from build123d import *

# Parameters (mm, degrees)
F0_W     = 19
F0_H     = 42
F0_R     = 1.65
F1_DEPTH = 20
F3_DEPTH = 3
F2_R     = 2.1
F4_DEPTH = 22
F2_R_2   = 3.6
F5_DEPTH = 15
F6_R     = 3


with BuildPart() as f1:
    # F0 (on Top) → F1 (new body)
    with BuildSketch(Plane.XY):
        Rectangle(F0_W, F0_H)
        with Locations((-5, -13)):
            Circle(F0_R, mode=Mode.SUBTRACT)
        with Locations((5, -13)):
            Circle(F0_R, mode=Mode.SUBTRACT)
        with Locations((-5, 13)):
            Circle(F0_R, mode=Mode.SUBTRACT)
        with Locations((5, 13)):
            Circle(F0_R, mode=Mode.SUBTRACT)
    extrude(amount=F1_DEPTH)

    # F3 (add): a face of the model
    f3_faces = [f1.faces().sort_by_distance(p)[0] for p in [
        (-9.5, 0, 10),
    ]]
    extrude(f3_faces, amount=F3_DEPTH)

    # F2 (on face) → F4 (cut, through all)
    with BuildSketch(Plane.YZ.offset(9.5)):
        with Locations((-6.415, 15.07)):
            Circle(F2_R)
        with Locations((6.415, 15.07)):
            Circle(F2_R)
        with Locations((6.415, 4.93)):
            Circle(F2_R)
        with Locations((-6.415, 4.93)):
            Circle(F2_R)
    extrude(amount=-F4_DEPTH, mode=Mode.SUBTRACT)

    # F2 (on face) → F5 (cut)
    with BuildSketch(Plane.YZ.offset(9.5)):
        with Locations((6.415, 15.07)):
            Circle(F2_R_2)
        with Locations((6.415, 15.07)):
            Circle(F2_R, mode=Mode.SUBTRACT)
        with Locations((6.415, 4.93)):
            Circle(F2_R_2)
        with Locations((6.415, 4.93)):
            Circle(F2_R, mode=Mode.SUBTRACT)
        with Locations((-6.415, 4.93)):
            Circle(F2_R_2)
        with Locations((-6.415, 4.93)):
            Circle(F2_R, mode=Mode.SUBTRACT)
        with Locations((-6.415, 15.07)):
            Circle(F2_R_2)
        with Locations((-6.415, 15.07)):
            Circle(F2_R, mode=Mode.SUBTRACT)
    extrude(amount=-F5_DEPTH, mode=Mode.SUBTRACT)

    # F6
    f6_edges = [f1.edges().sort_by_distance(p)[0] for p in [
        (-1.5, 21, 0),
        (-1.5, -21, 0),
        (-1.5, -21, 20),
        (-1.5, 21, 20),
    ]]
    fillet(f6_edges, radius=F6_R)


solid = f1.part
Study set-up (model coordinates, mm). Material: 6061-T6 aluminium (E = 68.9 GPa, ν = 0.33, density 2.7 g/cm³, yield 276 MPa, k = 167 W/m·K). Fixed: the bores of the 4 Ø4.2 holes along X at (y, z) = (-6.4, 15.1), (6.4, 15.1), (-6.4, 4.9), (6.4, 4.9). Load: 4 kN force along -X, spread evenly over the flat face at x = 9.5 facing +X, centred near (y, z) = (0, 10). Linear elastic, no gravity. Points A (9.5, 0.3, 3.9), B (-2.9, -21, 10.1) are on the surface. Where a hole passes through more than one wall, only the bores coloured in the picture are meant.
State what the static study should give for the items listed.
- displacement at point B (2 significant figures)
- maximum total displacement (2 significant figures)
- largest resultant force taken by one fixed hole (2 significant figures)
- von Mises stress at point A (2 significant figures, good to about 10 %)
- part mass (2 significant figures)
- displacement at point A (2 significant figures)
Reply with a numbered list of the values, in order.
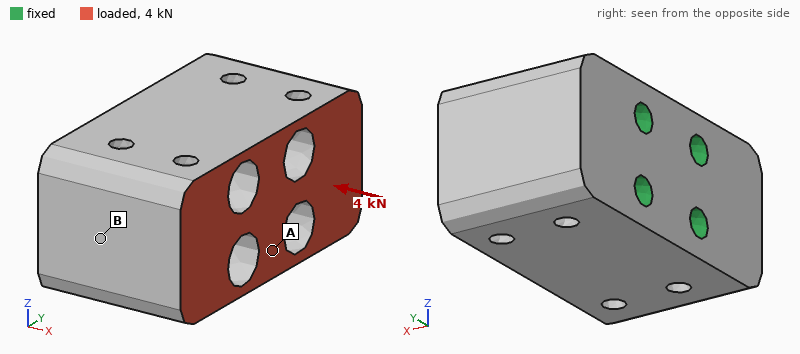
1. 4.5 µm
2. 5.7 µm
3. 1.0 kN
4. 8.7 MPa
5. 40 g
6. 2.3 µm
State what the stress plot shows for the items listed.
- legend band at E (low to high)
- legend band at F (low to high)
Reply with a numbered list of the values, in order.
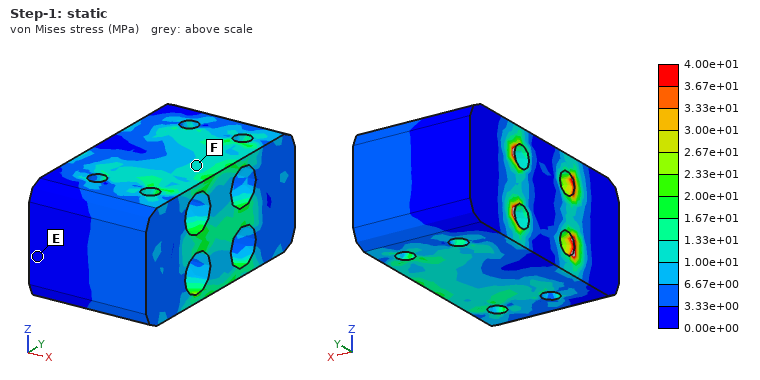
1. 0.00e+00 to 3.33e+00 MPa
2. 1.00e+01 to 1.33e+01 MPa
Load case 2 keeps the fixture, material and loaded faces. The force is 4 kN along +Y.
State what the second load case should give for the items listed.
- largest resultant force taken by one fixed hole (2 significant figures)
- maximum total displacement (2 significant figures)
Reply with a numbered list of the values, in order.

1. 2.1 kN
2. 29 µm
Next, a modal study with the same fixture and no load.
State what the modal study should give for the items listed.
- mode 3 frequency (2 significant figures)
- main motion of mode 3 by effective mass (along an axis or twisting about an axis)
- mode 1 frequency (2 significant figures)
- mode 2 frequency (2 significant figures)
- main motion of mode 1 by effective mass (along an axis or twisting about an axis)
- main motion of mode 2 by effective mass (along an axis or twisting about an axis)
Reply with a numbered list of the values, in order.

1. 21 kHz
2. twisting about X
3. 16 kHz
4. 19 kHz
5. along Y
6. along Z
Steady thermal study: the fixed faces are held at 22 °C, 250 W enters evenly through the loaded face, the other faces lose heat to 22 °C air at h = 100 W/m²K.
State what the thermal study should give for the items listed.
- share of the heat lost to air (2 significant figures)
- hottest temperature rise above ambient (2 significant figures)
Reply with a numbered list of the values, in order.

1. 6.0 %
2. 56 K
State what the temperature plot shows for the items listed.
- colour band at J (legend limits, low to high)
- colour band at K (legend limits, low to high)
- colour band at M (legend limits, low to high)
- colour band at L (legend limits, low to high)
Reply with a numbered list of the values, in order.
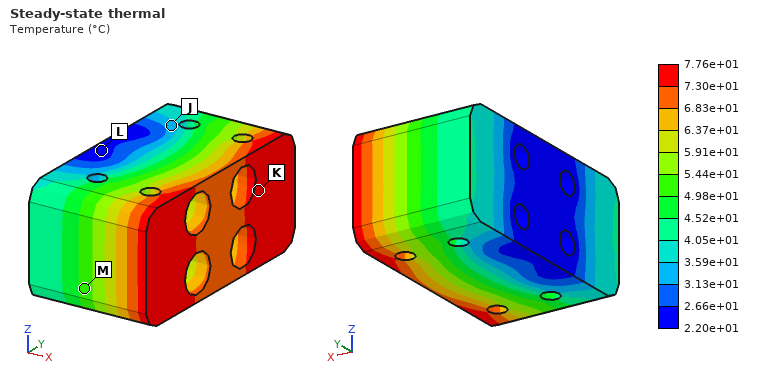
1. 3.13e+01 to 3.59e+01 °C
2. 7.30e+01 to 7.76e+01 °C
3. 4.98e+01 to 5.44e+01 °C
4. 2.20e+01 to 2.66e+01 °C
